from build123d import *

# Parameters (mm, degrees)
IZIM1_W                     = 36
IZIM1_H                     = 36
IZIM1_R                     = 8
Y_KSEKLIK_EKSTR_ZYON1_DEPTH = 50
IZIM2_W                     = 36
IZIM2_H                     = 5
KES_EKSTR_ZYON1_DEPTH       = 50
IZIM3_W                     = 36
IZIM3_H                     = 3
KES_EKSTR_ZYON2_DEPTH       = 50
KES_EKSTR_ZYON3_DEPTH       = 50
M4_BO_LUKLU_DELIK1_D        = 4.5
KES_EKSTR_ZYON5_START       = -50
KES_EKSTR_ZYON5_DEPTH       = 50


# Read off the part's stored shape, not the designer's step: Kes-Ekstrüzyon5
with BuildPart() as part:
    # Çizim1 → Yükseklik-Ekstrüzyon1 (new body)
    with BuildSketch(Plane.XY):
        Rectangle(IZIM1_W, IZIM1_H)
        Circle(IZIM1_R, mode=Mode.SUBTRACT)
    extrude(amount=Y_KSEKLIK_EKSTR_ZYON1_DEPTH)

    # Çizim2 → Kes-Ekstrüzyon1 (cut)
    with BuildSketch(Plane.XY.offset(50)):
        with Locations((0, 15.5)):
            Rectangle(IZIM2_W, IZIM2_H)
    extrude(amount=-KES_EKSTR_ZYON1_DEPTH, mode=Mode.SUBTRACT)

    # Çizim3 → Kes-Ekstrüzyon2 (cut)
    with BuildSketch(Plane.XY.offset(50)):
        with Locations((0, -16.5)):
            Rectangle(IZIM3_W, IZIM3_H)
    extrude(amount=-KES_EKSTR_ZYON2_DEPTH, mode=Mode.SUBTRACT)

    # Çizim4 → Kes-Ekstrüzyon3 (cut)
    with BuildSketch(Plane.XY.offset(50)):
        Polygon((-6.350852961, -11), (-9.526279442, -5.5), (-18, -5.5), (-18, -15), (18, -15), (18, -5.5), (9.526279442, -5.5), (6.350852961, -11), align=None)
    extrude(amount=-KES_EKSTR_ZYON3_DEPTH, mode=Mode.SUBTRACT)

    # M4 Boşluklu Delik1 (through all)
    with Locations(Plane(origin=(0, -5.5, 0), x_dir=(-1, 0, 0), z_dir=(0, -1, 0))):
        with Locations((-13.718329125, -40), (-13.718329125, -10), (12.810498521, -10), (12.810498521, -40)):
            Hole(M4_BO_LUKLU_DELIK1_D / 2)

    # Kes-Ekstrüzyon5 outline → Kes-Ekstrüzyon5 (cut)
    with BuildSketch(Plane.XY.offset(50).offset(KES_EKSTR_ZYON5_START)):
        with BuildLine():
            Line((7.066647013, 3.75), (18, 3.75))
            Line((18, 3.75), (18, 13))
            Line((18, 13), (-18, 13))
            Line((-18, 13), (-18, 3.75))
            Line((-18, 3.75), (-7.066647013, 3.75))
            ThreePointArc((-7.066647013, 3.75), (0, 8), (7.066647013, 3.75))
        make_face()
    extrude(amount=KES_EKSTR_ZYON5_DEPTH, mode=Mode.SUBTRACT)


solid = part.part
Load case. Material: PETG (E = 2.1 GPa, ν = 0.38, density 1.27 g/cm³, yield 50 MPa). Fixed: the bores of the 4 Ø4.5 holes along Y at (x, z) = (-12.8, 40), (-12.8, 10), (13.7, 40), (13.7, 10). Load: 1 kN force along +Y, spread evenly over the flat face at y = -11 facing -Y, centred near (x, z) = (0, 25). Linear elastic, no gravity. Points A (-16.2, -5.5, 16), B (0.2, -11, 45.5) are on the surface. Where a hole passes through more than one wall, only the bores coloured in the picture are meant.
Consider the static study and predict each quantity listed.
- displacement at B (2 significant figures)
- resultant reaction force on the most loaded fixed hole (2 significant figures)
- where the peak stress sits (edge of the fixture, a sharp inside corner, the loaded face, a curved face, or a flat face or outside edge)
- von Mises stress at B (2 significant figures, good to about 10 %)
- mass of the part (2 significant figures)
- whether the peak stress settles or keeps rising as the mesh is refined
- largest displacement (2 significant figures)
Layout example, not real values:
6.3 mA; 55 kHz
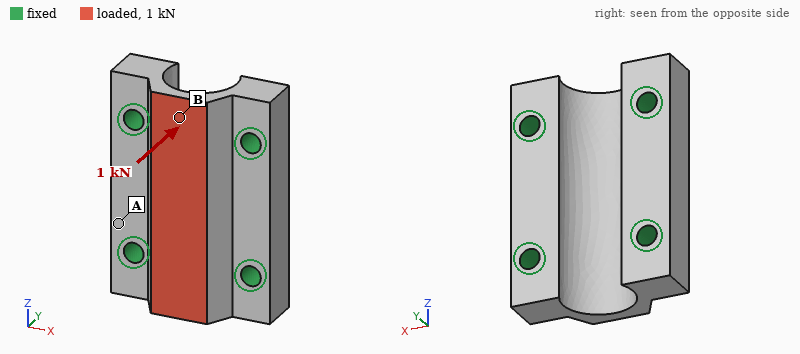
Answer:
56 µm; 330 N; edge of the fixture; 6.7 MPa; 16 g; keeps rising; 65 µm
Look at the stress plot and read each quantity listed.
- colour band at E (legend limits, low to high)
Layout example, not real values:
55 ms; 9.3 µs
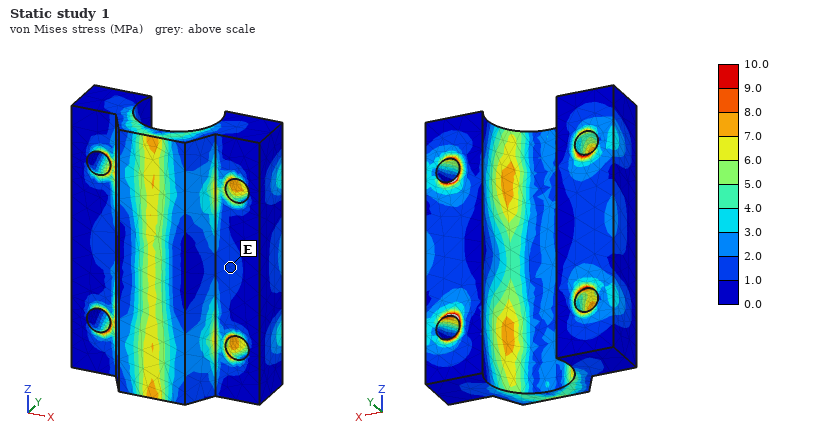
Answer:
1.0 to 2.0 MPa
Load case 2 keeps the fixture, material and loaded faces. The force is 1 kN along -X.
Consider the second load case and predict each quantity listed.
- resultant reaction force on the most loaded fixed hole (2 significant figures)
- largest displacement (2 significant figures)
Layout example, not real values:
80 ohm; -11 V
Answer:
300 N; 53 µm
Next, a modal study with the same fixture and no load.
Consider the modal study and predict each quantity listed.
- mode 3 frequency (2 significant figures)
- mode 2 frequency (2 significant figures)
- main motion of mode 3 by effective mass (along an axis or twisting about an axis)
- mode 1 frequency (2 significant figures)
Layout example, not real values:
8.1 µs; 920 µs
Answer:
9500 Hz; 9100 Hz; along Z; 8900 Hz
